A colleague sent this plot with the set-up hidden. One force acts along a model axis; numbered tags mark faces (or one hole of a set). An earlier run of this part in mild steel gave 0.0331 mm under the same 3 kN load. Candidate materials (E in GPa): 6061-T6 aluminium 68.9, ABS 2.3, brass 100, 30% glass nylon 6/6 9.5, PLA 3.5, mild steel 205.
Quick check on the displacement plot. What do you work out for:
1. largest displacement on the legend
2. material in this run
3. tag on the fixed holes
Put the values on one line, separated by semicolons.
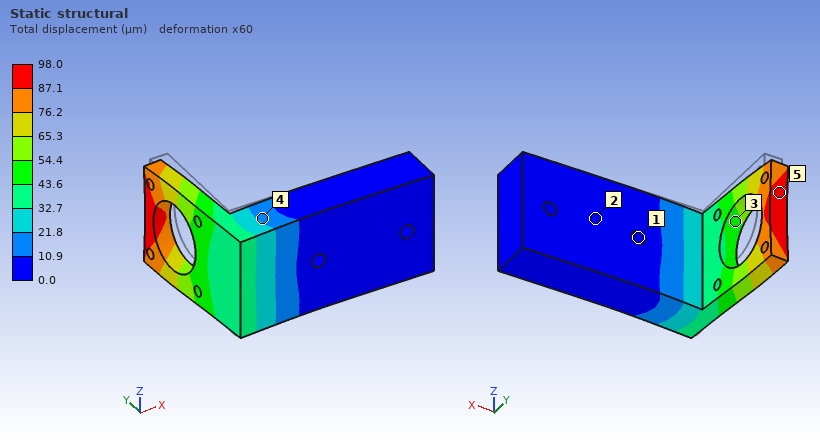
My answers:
98.0 µm; 6061-T6 aluminium; 1
